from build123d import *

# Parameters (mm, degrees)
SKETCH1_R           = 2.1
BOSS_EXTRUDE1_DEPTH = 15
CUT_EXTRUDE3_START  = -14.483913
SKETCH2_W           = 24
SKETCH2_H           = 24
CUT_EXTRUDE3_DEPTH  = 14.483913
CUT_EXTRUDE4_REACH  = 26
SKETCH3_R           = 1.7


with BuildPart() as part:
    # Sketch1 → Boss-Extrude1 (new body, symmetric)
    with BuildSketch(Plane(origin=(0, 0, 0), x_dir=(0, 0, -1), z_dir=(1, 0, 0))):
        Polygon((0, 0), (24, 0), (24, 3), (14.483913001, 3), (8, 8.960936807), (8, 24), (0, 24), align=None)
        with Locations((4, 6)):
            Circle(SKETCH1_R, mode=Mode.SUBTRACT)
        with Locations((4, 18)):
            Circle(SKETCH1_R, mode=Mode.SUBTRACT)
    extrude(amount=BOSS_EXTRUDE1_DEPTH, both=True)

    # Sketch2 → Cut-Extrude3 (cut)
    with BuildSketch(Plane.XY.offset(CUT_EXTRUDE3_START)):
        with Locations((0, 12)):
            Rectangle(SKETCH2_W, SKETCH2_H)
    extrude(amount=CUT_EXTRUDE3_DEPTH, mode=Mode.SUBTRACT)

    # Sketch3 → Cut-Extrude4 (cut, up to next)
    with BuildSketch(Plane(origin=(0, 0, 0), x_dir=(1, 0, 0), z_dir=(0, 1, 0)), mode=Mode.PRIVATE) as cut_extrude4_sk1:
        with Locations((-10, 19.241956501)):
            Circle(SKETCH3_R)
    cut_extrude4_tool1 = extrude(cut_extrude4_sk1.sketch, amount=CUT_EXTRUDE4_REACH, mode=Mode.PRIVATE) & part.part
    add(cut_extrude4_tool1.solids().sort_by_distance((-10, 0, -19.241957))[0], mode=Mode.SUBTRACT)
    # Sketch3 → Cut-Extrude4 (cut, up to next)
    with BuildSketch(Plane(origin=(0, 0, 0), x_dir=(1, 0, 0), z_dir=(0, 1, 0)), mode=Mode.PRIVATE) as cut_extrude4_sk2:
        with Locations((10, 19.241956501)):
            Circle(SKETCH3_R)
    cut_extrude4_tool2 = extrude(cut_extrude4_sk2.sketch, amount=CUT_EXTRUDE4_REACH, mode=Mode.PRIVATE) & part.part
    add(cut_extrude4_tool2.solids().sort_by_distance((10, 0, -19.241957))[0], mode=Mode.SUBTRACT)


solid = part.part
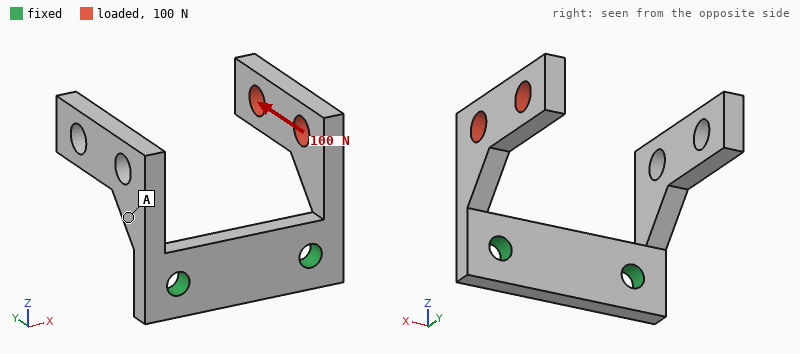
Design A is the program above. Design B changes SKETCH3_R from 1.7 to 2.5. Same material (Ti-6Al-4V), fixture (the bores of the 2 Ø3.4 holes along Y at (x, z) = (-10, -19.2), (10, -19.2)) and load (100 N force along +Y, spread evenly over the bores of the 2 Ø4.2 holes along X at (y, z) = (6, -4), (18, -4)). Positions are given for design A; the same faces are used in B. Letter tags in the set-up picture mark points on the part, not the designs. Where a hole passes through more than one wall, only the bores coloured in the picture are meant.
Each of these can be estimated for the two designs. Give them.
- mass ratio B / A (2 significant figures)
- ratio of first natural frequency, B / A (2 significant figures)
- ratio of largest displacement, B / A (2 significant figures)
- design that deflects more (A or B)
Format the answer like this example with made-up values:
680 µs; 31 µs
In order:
0.97; 1.0; 0.89; A
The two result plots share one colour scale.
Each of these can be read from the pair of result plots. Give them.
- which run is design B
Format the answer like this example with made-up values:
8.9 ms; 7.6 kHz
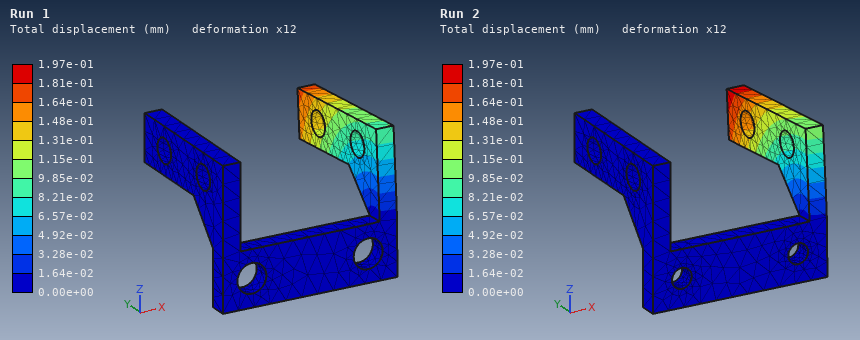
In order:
Run 1
